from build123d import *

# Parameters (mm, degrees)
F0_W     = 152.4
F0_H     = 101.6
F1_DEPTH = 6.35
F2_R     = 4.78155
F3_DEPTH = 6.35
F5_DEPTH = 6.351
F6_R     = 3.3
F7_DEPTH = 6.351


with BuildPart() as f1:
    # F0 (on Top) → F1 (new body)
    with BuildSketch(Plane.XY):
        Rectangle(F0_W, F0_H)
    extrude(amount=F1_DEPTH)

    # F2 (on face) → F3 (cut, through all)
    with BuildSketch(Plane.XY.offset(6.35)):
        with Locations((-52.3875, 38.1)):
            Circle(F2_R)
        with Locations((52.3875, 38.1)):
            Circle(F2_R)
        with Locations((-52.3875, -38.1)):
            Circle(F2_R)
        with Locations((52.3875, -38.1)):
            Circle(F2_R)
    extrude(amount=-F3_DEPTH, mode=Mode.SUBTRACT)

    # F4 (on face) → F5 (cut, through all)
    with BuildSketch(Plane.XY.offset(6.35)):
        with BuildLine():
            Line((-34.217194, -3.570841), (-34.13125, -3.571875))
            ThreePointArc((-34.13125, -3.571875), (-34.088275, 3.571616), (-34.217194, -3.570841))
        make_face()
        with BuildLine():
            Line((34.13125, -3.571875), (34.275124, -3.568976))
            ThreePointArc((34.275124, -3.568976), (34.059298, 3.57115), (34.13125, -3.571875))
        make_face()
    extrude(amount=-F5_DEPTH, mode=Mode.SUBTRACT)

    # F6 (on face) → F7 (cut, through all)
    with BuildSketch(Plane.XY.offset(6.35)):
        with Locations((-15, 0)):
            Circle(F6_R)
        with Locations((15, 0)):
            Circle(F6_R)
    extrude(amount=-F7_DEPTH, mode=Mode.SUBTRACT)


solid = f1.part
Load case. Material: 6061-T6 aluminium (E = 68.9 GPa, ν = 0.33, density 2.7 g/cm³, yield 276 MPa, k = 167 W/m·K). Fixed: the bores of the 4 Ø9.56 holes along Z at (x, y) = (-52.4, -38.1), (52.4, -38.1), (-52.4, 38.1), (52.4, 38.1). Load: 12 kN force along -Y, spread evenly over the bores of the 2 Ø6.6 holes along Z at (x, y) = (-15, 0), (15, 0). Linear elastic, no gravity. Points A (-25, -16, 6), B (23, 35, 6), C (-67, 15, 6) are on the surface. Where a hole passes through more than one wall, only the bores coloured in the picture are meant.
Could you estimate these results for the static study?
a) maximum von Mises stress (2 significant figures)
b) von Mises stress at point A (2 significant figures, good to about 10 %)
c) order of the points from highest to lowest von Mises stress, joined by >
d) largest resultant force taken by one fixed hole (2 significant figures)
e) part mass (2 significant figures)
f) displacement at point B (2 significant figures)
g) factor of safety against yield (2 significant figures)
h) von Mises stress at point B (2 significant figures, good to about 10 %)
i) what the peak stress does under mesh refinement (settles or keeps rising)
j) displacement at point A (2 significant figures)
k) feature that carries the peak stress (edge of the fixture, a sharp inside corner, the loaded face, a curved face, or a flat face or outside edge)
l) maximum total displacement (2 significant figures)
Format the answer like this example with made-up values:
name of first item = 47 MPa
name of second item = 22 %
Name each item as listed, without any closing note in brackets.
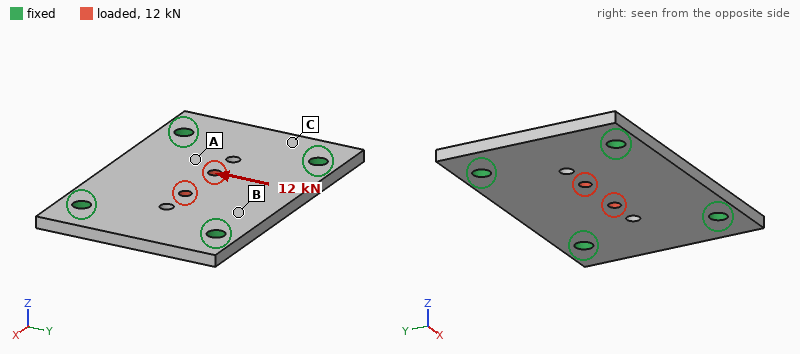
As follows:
maximum von Mises stress = 80 MPa
von Mises stress at point A = 22 MPa
order of the points from highest to lowest von Mises stress, joined by > = A > B > C
largest resultant force taken by one fixed hole = 3.5 kN
part mass = 260 g
displacement at point B = 14 µm
factor of safety against yield = 3.4
von Mises stress at point B = 13 MPa
what the peak stress does under mesh refinement = settles
displacement at point A = 14 µm
feature that carries the peak stress = the loaded face
maximum total displacement = 24 µm
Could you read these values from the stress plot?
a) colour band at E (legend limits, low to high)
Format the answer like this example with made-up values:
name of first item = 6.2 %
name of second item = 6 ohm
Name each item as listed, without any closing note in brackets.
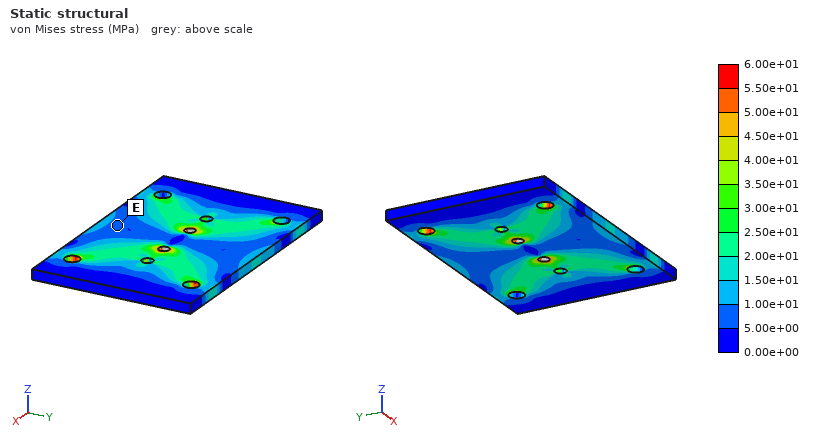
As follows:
colour band at E = 5.00e+00 to 1.00e+01 MPa
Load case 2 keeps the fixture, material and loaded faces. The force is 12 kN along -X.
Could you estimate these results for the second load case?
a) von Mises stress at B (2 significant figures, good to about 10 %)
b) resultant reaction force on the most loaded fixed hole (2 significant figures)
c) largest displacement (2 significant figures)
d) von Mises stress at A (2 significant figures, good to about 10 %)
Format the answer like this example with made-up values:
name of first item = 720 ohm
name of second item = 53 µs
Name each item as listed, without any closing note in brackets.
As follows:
von Mises stress at B = 8.7 MPa
resultant reaction force on the most loaded fixed hole = 3.1 kN
largest displacement = 20 µm
von Mises stress at A = 16 MPa
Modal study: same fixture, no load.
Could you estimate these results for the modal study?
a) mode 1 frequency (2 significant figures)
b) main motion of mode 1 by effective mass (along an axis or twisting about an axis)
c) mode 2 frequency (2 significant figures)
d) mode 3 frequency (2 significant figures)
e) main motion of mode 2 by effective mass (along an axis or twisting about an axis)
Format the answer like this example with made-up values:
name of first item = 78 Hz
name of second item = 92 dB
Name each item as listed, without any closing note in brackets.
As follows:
mode 1 frequency = 2700 Hz
main motion of mode 1 by effective mass = along Z
mode 2 frequency = 3800 Hz
mode 3 frequency = 5100 Hz
main motion of mode 2 by effective mass = twisting about X
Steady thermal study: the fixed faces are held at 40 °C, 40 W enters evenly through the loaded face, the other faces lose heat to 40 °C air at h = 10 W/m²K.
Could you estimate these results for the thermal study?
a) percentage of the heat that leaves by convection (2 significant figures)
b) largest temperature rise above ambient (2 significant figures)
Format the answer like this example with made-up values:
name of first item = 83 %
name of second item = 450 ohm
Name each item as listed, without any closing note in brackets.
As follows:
percentage of the heat that leaves by convection = 3.7 %
largest temperature rise above ambient = 15 K
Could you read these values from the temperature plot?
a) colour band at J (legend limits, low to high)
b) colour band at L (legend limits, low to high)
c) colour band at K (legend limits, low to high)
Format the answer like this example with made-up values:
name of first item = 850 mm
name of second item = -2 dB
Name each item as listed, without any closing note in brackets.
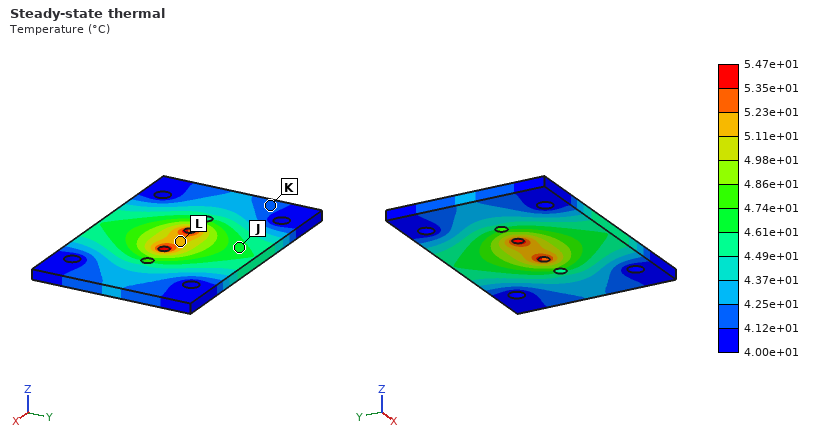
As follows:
colour band at J = 4.61e+01 to 4.74e+01 °C
colour band at L = 5.11e+01 to 5.23e+01 °C
colour band at K = 4.12e+01 to 4.25e+01 °C
